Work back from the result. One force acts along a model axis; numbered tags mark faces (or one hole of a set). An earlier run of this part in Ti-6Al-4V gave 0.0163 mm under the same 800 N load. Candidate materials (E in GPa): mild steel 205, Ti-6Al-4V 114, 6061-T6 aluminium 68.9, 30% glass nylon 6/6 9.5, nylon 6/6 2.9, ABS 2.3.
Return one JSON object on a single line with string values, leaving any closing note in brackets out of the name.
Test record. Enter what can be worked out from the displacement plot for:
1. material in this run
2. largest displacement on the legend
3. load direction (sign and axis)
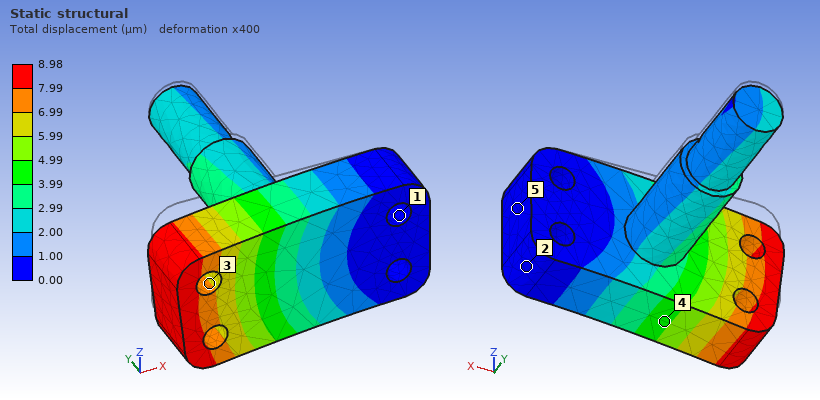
{"material in this run": "mild steel", "largest displacement on the legend": "8.98 µm", "load direction": "-Z"}
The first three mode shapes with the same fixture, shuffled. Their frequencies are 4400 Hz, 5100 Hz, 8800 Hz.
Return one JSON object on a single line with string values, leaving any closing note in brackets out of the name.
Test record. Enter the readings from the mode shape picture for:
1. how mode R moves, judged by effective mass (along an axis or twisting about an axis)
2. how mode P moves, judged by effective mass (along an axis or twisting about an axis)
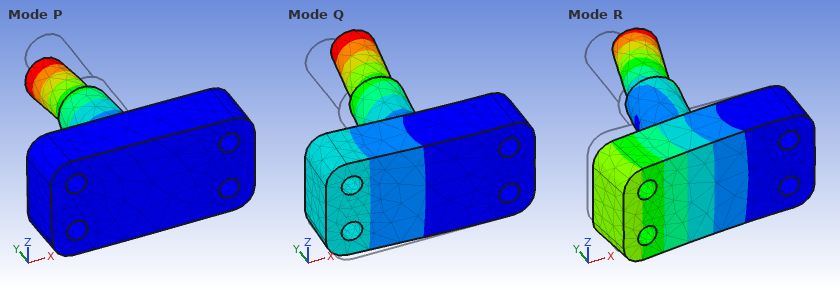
{"how mode R moves, judged by effective mass": "along Y", "how mode P moves, judged by effective mass": "along Z"}
